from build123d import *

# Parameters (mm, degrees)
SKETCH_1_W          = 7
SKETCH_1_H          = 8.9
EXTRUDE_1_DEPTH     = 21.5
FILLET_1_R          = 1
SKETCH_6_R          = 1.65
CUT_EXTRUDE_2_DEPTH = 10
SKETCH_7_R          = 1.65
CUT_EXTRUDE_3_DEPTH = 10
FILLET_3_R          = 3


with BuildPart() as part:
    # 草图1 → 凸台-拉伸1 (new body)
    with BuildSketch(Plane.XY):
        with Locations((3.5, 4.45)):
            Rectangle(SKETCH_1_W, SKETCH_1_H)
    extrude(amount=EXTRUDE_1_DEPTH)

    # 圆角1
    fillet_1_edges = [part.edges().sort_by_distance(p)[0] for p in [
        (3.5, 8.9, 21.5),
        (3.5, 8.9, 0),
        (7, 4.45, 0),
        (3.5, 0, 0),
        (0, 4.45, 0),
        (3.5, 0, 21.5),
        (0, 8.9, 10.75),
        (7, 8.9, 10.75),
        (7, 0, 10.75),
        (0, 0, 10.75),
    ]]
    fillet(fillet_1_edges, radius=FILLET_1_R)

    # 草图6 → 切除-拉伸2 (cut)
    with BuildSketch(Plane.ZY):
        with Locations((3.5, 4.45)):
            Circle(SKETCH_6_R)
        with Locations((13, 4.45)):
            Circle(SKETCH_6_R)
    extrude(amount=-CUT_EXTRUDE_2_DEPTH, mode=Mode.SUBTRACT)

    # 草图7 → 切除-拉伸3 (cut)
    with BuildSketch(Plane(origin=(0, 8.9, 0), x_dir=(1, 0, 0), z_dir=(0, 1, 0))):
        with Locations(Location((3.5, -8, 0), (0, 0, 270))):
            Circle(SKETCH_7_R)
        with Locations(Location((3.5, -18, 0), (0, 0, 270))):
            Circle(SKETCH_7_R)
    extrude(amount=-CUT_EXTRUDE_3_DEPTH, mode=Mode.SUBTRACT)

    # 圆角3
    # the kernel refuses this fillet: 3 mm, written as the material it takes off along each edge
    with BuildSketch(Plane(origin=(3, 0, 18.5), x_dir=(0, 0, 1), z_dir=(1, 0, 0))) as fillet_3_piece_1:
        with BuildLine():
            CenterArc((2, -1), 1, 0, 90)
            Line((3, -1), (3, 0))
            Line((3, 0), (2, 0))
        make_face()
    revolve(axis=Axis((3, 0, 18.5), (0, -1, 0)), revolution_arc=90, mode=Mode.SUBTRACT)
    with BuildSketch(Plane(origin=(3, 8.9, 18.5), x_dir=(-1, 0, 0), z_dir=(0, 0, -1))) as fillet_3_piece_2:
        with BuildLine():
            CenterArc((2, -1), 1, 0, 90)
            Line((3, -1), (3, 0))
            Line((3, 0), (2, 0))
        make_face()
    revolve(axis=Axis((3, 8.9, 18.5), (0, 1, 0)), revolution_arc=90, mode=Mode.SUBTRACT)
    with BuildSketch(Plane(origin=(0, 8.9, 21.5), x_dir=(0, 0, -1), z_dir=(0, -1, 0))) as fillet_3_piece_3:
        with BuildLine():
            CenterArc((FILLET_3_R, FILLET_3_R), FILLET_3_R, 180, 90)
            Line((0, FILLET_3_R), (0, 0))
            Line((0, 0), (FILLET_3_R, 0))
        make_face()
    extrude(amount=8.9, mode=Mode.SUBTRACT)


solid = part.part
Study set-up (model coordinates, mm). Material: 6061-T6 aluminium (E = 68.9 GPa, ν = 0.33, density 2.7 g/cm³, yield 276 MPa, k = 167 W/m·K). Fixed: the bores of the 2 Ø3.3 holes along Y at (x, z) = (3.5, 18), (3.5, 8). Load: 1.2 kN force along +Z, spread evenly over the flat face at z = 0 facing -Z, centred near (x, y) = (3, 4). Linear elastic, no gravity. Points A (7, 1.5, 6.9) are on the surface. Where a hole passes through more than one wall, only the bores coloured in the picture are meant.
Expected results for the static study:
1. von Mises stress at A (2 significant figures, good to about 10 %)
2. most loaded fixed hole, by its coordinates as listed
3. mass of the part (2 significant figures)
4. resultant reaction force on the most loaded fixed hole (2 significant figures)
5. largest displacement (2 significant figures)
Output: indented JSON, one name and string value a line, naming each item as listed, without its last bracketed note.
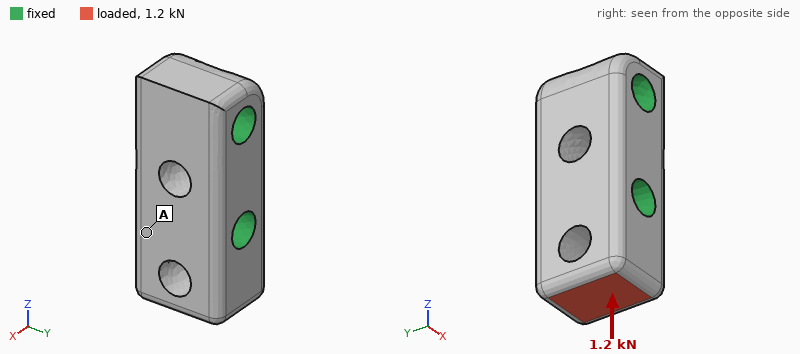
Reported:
{
  "von Mises stress at A": "16 MPa",
  "most loaded fixed hole, by its coordinates as listed": "(3.5, 8)",
  "mass of the part": "2.8 g",
  "resultant reaction force on the most loaded fixed hole": "1.2 kN",
  "largest displacement": "5.4 µm"
}
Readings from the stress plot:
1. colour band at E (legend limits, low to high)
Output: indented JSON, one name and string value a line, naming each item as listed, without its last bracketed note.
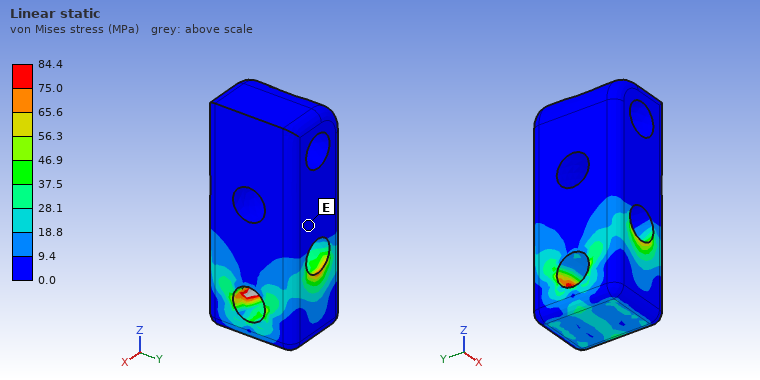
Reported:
{
  "colour band at E": "0.0 to 9.4 MPa"
}
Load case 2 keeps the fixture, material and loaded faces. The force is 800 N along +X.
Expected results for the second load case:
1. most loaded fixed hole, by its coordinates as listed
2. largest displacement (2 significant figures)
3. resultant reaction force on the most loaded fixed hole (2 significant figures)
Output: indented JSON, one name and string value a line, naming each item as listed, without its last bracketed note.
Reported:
{
  "most loaded fixed hole, by its coordinates as listed": "(3.5, 8)",
  "largest displacement": "19 µm",
  "resultant reaction force on the most loaded fixed hole": "910 N"
}
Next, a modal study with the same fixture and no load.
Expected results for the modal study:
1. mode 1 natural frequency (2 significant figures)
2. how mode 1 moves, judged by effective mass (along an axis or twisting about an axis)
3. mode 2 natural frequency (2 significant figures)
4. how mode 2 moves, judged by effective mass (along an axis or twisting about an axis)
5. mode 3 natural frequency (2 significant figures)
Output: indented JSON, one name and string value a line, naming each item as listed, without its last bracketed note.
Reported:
{
  "mode 1 natural frequency": "60 kHz",
  "how mode 1 moves, judged by effective mass": "along X",
  "mode 2 natural frequency": "69 kHz",
  "how mode 2 moves, judged by effective mass": "along Y",
  "mode 3 natural frequency": "90 kHz"
}
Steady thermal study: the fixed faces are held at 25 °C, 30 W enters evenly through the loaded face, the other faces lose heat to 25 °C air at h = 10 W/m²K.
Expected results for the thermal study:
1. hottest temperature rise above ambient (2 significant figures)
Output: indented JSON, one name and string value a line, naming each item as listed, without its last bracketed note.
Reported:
{
  "hottest temperature rise above ambient": "32 K"
}
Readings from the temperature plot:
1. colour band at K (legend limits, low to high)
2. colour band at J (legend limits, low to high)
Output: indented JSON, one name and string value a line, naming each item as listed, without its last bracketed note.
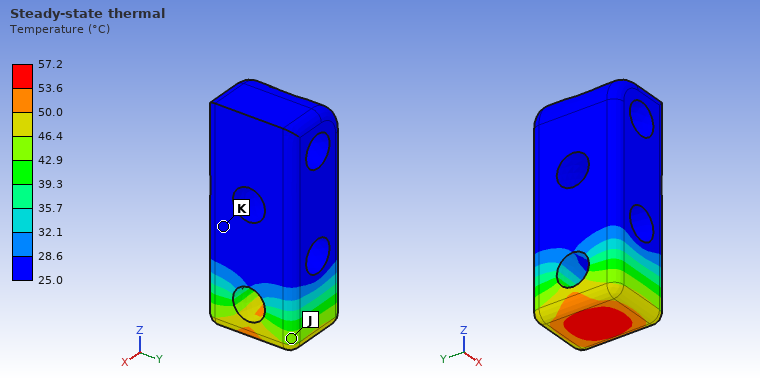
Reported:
{
  "colour band at K": "25.0 to 28.6 °C",
  "colour band at J": "42.9 to 46.4 °C"
}
